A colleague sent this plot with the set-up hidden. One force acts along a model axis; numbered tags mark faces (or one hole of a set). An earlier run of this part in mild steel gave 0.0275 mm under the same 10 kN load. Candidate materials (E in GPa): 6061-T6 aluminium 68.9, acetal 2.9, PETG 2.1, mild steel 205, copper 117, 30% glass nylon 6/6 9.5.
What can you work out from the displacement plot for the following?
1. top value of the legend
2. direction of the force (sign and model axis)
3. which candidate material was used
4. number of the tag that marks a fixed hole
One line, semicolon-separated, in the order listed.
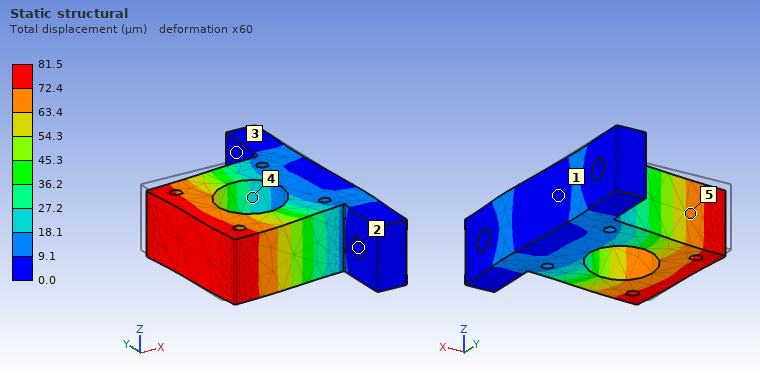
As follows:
81.5 µm; -Y; 6061-T6 aluminium; 2
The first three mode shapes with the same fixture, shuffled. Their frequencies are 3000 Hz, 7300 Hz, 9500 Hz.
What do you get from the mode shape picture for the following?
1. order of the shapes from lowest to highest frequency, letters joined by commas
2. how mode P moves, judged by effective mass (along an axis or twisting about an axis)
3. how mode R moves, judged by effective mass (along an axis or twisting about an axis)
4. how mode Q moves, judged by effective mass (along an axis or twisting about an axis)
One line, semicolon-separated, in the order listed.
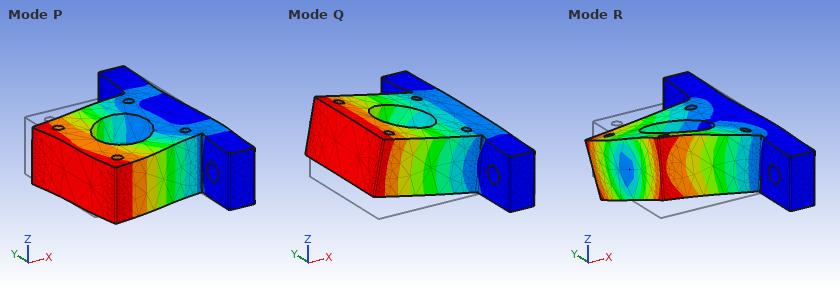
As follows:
Q, P, R; along Y; twisting about X; along Z
